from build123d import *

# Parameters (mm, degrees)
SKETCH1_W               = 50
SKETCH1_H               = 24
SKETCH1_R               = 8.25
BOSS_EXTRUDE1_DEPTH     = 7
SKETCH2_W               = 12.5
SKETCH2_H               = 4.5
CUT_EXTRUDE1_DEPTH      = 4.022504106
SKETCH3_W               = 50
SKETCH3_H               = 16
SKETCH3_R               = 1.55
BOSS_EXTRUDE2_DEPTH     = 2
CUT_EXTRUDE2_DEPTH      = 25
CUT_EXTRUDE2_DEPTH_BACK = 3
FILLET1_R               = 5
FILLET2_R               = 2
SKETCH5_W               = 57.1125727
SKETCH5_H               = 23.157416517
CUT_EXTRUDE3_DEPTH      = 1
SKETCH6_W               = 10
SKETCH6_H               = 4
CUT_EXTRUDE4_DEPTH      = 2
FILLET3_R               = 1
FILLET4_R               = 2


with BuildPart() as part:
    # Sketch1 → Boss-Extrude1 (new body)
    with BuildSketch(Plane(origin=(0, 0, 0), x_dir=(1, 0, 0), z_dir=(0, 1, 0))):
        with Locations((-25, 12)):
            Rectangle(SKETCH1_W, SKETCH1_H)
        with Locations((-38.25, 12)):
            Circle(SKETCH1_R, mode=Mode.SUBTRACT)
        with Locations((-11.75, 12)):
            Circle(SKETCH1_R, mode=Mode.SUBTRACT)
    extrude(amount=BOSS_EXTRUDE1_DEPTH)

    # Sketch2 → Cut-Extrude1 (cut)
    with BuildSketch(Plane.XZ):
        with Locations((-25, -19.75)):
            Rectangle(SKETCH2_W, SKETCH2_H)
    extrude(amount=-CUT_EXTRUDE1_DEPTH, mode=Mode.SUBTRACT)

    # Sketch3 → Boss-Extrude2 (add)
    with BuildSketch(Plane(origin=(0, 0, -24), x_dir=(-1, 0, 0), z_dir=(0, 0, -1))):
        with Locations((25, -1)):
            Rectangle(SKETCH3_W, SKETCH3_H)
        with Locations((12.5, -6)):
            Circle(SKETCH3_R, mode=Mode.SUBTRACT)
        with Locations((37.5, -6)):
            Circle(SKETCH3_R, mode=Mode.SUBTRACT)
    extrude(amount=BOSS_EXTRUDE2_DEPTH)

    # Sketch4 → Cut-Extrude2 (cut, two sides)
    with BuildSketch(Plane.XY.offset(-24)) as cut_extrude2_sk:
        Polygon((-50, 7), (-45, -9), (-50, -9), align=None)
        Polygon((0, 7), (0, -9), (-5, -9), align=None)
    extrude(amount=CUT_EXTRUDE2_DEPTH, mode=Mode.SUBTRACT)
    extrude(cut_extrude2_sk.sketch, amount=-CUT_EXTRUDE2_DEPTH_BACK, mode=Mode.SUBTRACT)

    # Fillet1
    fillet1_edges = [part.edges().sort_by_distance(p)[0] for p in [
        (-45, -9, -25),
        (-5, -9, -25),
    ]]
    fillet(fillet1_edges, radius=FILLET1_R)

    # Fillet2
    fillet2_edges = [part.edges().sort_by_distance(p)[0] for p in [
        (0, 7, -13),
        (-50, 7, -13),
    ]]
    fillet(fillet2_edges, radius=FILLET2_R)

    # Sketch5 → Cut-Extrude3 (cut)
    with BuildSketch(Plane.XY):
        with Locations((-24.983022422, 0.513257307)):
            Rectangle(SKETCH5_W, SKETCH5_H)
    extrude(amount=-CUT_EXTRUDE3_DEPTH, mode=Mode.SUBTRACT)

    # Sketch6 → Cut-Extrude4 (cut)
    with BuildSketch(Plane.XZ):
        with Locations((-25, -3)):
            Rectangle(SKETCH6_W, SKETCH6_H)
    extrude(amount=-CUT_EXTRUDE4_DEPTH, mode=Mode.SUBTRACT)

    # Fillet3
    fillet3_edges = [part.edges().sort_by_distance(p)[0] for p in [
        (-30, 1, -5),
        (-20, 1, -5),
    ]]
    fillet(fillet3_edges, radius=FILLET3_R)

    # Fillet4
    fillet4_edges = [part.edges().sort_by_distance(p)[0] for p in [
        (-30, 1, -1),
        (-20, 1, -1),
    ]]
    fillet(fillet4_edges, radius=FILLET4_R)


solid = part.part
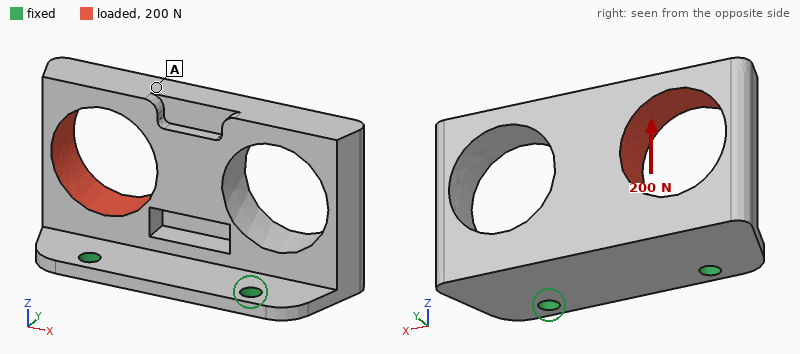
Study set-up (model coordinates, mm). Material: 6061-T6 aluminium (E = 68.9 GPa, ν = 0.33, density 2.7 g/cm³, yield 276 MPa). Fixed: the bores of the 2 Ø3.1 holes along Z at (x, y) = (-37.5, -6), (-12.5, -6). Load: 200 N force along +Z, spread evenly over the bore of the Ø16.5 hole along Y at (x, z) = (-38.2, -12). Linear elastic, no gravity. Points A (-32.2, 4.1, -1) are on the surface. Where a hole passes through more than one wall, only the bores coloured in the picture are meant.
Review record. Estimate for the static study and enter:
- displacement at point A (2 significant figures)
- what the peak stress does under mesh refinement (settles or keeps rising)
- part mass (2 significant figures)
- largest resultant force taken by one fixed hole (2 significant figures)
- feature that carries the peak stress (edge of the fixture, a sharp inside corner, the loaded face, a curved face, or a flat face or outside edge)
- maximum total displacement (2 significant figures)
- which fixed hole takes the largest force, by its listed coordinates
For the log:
0.13 mm
keeps rising
15 g
200 N
edge of the fixture
0.14 mm
(-37.5, -6)
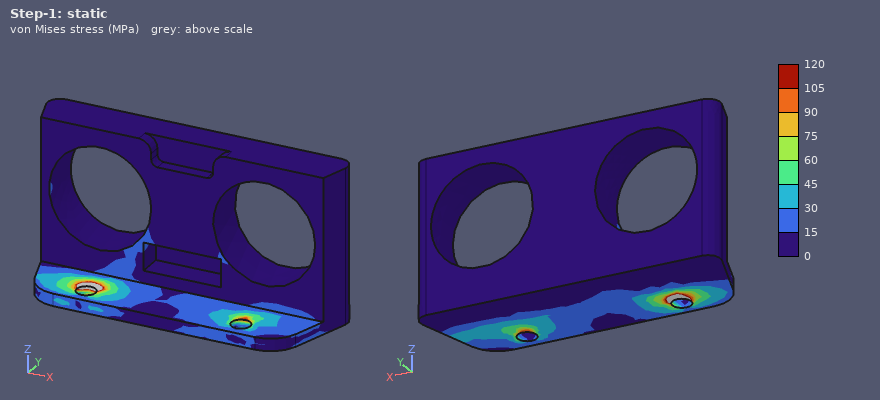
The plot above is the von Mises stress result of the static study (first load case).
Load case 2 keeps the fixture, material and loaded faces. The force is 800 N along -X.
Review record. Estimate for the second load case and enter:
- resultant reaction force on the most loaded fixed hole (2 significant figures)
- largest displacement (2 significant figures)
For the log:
620 N
0.10 mm
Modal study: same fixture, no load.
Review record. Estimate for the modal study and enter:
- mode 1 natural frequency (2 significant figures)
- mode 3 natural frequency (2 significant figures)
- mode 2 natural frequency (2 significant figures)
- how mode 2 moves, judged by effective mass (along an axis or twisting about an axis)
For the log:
1400 Hz
7400 Hz
4100 Hz
along X
